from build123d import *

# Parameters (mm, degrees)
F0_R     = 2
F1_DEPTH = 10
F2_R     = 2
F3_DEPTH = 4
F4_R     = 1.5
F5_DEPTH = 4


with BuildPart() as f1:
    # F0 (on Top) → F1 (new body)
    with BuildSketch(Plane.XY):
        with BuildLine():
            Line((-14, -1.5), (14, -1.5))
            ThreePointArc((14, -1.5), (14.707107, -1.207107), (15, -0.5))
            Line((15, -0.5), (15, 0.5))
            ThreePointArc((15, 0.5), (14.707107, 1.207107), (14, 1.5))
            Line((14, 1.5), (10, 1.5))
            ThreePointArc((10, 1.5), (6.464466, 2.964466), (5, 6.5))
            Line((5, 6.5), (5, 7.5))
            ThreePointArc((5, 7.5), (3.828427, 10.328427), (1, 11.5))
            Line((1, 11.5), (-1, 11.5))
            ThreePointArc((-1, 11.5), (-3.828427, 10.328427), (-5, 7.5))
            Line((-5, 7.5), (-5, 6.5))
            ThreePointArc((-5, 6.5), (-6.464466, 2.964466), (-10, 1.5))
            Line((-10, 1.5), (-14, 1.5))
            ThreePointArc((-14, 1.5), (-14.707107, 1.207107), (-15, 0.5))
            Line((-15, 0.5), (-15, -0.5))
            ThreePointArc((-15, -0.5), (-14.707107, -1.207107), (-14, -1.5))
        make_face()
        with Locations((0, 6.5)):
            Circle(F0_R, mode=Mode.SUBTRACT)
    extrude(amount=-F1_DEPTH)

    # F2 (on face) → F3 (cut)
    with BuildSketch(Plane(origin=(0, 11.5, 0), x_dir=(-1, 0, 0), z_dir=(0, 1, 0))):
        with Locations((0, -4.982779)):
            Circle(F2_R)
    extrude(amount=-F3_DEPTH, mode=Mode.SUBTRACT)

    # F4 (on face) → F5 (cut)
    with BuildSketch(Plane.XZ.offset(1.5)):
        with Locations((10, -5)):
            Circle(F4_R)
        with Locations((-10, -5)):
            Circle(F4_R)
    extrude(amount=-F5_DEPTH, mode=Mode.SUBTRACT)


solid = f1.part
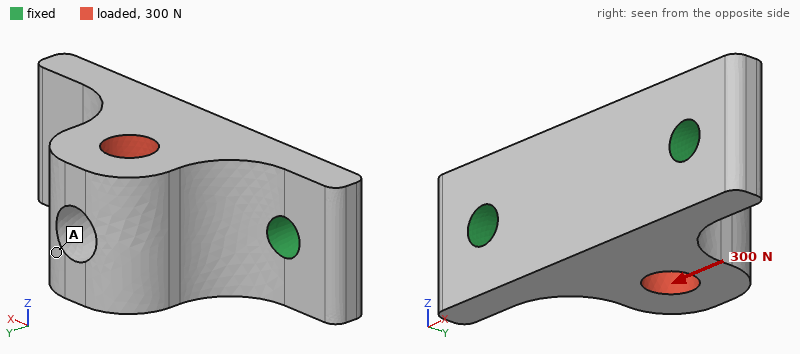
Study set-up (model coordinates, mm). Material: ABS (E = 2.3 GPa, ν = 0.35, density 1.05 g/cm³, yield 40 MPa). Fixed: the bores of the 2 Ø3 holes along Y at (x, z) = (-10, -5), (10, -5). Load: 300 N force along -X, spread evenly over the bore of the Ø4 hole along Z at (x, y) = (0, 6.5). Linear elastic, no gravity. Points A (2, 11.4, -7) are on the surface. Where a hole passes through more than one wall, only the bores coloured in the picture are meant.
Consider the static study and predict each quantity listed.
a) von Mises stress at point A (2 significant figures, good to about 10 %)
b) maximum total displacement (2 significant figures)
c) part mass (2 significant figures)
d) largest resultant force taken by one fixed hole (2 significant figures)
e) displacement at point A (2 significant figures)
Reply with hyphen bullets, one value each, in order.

- 2.4 MPa
- 73 µm
- 1.8 g
- 180 N
- 70 µm
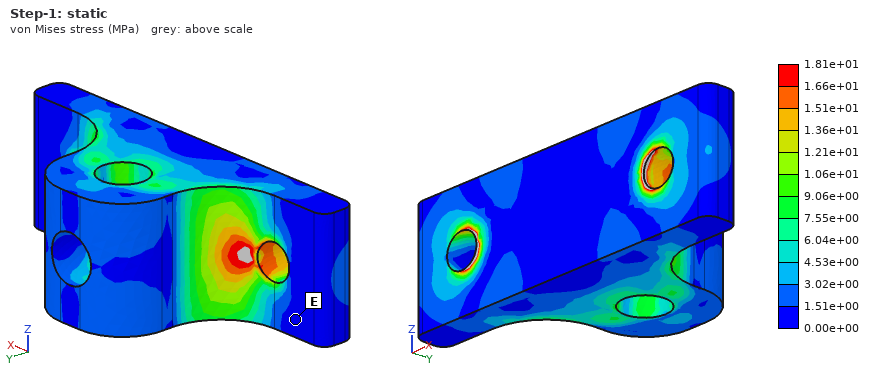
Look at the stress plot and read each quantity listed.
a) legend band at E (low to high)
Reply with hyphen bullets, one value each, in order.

- 0.00e+00 to 1.51e+00 MPa
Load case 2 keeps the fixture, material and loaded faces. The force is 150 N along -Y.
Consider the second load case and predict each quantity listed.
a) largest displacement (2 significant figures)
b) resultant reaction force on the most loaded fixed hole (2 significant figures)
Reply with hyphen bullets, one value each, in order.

- 31 µm
- 88 N
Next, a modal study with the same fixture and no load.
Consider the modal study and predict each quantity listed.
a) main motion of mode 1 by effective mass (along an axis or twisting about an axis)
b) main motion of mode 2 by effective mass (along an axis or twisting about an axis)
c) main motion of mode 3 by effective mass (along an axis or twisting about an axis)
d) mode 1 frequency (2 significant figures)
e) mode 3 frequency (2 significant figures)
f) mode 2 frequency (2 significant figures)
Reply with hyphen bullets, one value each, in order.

- along Z
- along Y
- along X
- 5100 Hz
- 13 kHz
- 11 kHz
